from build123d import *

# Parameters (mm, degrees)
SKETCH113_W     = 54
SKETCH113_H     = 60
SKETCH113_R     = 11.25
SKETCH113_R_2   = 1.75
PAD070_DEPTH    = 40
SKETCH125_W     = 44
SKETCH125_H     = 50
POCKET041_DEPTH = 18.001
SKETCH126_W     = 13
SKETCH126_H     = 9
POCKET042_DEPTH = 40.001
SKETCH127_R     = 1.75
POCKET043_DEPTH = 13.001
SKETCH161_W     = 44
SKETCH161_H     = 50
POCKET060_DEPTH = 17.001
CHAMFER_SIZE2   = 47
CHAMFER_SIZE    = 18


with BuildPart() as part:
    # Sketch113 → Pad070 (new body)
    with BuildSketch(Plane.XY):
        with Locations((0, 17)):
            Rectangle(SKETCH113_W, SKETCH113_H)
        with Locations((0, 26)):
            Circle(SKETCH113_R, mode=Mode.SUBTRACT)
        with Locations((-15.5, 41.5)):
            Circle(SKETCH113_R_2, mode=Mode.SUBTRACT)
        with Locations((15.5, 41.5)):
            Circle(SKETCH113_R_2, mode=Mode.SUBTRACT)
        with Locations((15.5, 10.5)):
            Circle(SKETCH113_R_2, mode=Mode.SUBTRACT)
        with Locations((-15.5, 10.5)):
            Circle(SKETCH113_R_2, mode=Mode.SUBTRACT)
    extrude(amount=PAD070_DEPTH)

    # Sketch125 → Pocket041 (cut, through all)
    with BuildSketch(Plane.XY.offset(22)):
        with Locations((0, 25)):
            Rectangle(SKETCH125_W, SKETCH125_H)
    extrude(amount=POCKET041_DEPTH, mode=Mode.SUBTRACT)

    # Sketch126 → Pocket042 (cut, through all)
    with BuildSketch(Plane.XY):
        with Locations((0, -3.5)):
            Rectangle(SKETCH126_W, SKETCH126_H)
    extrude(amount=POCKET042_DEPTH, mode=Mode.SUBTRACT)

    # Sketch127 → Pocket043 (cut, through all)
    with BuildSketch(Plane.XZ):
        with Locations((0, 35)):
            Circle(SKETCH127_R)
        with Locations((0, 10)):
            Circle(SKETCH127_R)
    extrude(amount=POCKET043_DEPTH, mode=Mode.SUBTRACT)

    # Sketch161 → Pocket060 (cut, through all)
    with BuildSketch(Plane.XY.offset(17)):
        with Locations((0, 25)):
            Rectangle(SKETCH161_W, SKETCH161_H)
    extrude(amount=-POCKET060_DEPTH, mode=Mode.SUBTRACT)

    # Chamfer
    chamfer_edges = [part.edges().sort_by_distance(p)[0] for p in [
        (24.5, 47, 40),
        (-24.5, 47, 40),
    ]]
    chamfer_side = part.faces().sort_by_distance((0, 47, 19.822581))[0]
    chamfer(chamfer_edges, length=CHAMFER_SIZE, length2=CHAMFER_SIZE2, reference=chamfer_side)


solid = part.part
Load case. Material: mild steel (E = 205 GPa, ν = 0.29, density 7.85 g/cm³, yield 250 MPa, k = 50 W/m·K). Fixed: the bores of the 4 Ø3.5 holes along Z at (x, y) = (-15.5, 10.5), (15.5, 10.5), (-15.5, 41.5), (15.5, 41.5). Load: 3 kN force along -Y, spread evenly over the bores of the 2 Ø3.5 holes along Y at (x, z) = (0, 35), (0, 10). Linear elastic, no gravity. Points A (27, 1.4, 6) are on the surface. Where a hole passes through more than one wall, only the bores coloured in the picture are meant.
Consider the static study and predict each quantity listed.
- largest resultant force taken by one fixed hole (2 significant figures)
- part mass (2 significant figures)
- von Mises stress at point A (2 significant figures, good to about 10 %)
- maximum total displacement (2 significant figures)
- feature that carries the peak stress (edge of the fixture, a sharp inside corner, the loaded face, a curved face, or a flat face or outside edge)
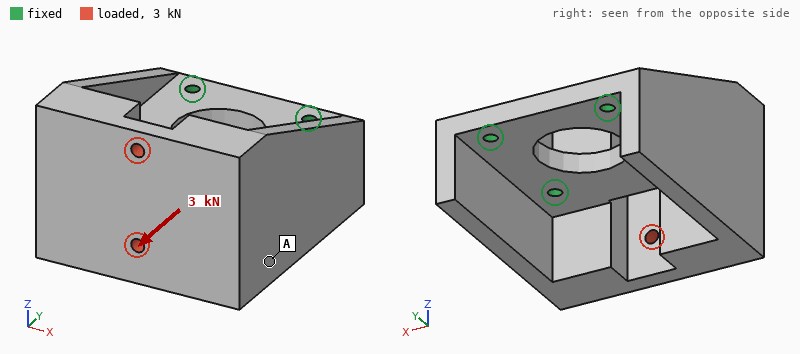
1.5 kN
360 g
9.3 MPa
10 µm
the loaded face
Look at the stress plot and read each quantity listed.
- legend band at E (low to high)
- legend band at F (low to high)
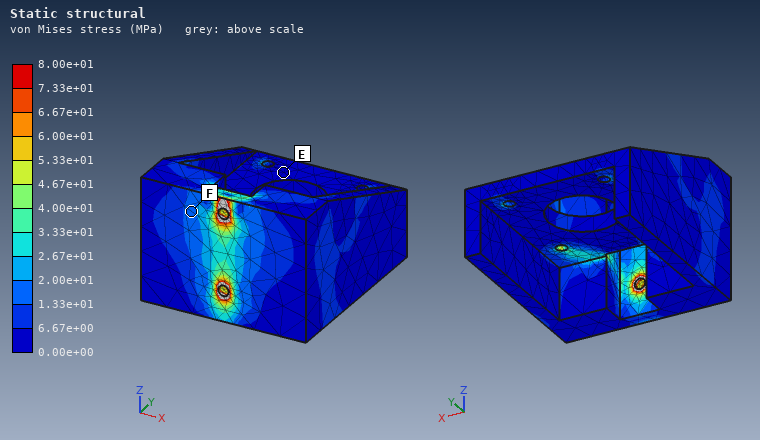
0.00e+00 to 6.67e+00 MPa
1.33e+01 to 2.00e+01 MPa
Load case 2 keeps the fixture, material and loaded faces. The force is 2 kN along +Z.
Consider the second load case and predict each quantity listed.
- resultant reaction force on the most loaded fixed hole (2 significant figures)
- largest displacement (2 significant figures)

1.5 kN
15 µm
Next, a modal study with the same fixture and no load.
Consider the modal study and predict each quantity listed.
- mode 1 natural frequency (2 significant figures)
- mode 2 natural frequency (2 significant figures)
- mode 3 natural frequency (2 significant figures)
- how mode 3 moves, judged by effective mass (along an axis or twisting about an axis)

4900 Hz
5000 Hz
7700 Hz
along Z
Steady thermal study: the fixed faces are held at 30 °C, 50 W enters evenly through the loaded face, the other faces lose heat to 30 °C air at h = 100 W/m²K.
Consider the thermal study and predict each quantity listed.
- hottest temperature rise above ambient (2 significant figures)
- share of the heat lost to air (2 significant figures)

73 K
55 %
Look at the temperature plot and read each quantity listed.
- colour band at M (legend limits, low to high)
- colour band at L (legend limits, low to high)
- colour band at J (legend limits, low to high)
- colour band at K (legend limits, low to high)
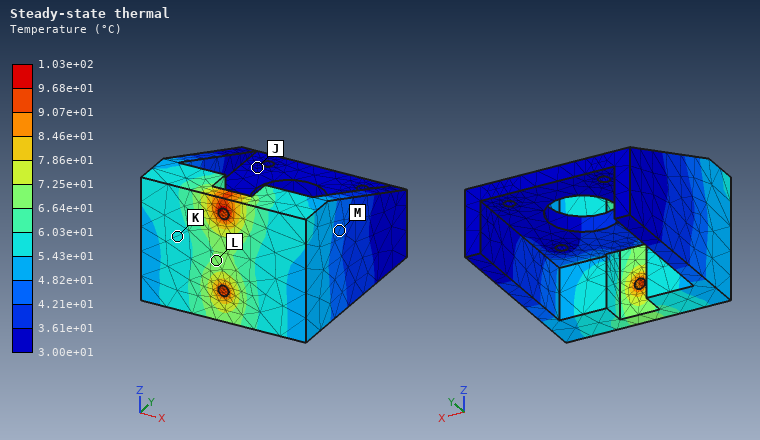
4.21e+01 to 4.82e+01 °C
6.64e+01 to 7.25e+01 °C
3.00e+01 to 3.61e+01 °C
5.43e+01 to 6.03e+01 °C
